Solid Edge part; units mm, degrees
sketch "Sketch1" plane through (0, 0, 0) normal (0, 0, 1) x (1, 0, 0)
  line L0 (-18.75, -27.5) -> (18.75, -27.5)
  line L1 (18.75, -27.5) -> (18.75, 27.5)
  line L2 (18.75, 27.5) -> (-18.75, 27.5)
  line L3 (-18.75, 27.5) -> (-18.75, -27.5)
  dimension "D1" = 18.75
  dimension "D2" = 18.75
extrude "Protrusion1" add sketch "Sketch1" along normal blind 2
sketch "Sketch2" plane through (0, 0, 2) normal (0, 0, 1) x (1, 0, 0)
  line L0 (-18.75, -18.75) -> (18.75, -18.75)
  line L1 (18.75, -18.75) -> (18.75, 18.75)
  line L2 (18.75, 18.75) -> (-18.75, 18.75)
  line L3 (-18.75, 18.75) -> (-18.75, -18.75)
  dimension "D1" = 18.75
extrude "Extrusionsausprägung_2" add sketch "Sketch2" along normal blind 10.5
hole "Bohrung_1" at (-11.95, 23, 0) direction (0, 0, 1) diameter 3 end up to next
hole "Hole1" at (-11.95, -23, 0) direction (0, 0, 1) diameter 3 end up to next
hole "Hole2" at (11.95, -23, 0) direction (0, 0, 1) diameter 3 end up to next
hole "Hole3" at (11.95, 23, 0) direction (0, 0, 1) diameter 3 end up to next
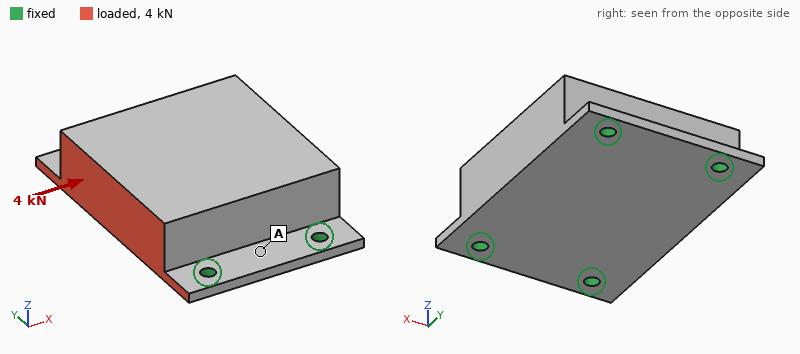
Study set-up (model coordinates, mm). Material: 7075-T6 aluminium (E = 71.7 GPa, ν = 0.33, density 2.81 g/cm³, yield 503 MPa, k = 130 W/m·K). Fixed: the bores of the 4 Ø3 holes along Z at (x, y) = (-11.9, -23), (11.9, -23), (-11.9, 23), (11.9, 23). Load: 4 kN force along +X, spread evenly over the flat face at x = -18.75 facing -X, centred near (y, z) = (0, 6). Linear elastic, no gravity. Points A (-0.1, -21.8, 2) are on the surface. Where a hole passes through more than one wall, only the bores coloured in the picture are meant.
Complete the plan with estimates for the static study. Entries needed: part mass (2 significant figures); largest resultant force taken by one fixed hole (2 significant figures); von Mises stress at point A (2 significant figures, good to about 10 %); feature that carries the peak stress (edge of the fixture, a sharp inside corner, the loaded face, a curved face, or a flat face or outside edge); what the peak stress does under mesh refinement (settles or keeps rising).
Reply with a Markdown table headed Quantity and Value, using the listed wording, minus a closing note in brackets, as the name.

| Quantity | Value |
|---|---|
| part mass | 53 g |
| largest resultant force taken by one fixed hole | 1.2 kN |
| von Mises stress at point A | 37 MPa |
| feature that carries the peak stress | edge of the fixture |
| what the peak stress does under mesh refinement | keeps rising |
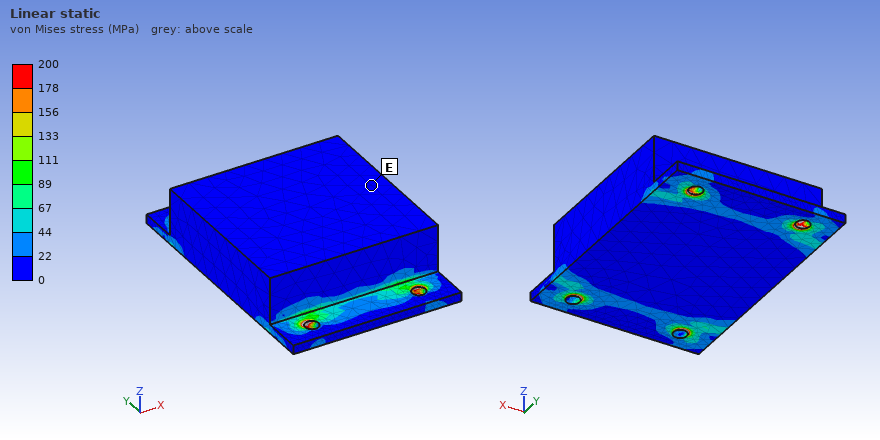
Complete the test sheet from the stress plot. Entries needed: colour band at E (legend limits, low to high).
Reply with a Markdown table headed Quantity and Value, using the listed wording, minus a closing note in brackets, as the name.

| Quantity | Value |
|---|---|
| colour band at E | 0 to 22 MPa |
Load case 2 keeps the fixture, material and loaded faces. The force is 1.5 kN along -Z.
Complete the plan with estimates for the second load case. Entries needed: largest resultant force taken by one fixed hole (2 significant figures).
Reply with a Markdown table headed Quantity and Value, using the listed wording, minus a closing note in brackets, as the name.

| Quantity | Value |
|---|---|
| largest resultant force taken by one fixed hole | 1.1 kN |
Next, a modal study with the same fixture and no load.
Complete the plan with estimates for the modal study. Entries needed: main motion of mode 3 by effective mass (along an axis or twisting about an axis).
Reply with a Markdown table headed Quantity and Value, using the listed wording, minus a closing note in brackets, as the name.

| Quantity | Value |
|---|---|
| main motion of mode 3 by effective mass | along Y |
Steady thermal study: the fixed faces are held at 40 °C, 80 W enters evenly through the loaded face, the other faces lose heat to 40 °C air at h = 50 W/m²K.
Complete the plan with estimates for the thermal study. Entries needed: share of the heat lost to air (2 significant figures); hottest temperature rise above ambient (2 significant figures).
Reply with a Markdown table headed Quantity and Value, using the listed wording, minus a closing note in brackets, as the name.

| Quantity | Value |
|---|---|
| share of the heat lost to air | 9.1 % |
| hottest temperature rise above ambient | 49 K |
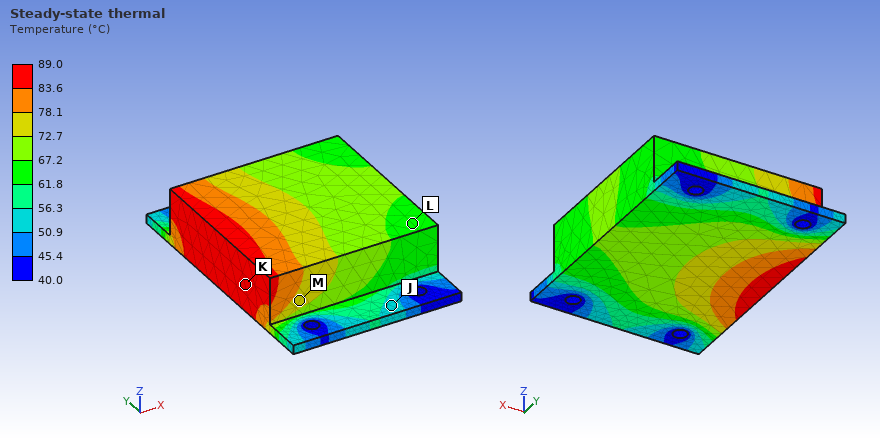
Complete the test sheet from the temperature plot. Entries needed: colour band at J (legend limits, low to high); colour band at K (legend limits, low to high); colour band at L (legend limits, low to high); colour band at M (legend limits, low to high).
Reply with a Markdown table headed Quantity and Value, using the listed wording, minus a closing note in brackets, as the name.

| Quantity | Value |
|---|---|
| colour band at J | 50.9 to 56.3 °C |
| colour band at K | 83.6 to 89.0 °C |
| colour band at L | 61.8 to 67.2 °C |
| colour band at M | 72.7 to 78.1 °C |
